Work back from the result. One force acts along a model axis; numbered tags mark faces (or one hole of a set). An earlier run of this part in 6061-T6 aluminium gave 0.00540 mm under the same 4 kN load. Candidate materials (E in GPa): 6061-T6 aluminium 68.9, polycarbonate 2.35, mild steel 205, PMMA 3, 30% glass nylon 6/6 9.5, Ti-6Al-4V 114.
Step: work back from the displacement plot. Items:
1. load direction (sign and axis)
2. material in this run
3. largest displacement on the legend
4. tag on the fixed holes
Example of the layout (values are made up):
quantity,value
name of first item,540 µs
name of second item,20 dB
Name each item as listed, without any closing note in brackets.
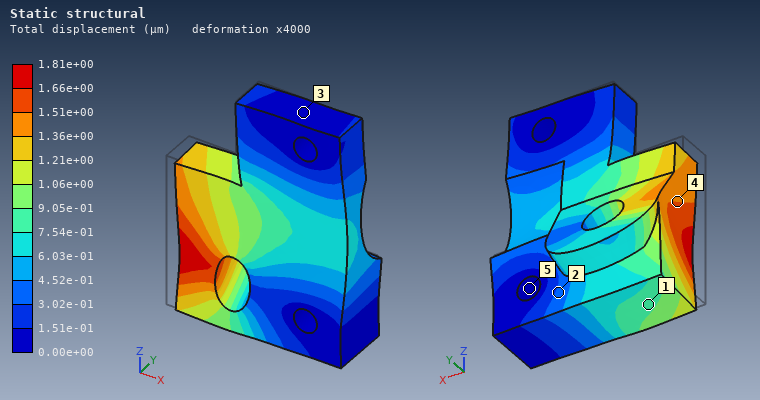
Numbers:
quantity,value
load direction,+X
material in this run,mild steel
largest displacement on the legend,1.81e+00 µm
tag on the fixed holes,5
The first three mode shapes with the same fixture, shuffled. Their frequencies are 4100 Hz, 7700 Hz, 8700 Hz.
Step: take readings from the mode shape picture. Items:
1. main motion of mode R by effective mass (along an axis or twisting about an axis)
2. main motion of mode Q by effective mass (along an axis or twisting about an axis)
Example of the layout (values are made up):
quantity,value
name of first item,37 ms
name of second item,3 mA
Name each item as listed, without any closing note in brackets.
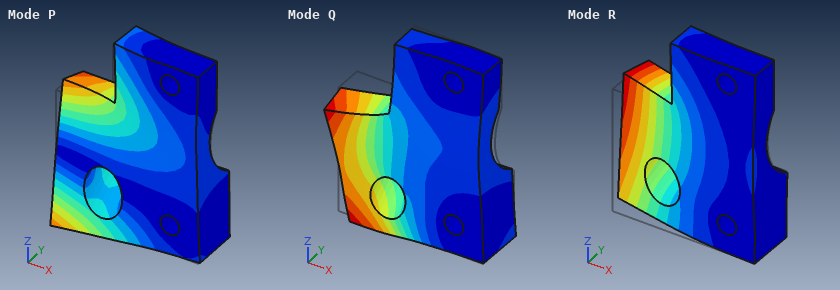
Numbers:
quantity,value
main motion of mode R by effective mass,along Y
main motion of mode Q by effective mass,along Z
